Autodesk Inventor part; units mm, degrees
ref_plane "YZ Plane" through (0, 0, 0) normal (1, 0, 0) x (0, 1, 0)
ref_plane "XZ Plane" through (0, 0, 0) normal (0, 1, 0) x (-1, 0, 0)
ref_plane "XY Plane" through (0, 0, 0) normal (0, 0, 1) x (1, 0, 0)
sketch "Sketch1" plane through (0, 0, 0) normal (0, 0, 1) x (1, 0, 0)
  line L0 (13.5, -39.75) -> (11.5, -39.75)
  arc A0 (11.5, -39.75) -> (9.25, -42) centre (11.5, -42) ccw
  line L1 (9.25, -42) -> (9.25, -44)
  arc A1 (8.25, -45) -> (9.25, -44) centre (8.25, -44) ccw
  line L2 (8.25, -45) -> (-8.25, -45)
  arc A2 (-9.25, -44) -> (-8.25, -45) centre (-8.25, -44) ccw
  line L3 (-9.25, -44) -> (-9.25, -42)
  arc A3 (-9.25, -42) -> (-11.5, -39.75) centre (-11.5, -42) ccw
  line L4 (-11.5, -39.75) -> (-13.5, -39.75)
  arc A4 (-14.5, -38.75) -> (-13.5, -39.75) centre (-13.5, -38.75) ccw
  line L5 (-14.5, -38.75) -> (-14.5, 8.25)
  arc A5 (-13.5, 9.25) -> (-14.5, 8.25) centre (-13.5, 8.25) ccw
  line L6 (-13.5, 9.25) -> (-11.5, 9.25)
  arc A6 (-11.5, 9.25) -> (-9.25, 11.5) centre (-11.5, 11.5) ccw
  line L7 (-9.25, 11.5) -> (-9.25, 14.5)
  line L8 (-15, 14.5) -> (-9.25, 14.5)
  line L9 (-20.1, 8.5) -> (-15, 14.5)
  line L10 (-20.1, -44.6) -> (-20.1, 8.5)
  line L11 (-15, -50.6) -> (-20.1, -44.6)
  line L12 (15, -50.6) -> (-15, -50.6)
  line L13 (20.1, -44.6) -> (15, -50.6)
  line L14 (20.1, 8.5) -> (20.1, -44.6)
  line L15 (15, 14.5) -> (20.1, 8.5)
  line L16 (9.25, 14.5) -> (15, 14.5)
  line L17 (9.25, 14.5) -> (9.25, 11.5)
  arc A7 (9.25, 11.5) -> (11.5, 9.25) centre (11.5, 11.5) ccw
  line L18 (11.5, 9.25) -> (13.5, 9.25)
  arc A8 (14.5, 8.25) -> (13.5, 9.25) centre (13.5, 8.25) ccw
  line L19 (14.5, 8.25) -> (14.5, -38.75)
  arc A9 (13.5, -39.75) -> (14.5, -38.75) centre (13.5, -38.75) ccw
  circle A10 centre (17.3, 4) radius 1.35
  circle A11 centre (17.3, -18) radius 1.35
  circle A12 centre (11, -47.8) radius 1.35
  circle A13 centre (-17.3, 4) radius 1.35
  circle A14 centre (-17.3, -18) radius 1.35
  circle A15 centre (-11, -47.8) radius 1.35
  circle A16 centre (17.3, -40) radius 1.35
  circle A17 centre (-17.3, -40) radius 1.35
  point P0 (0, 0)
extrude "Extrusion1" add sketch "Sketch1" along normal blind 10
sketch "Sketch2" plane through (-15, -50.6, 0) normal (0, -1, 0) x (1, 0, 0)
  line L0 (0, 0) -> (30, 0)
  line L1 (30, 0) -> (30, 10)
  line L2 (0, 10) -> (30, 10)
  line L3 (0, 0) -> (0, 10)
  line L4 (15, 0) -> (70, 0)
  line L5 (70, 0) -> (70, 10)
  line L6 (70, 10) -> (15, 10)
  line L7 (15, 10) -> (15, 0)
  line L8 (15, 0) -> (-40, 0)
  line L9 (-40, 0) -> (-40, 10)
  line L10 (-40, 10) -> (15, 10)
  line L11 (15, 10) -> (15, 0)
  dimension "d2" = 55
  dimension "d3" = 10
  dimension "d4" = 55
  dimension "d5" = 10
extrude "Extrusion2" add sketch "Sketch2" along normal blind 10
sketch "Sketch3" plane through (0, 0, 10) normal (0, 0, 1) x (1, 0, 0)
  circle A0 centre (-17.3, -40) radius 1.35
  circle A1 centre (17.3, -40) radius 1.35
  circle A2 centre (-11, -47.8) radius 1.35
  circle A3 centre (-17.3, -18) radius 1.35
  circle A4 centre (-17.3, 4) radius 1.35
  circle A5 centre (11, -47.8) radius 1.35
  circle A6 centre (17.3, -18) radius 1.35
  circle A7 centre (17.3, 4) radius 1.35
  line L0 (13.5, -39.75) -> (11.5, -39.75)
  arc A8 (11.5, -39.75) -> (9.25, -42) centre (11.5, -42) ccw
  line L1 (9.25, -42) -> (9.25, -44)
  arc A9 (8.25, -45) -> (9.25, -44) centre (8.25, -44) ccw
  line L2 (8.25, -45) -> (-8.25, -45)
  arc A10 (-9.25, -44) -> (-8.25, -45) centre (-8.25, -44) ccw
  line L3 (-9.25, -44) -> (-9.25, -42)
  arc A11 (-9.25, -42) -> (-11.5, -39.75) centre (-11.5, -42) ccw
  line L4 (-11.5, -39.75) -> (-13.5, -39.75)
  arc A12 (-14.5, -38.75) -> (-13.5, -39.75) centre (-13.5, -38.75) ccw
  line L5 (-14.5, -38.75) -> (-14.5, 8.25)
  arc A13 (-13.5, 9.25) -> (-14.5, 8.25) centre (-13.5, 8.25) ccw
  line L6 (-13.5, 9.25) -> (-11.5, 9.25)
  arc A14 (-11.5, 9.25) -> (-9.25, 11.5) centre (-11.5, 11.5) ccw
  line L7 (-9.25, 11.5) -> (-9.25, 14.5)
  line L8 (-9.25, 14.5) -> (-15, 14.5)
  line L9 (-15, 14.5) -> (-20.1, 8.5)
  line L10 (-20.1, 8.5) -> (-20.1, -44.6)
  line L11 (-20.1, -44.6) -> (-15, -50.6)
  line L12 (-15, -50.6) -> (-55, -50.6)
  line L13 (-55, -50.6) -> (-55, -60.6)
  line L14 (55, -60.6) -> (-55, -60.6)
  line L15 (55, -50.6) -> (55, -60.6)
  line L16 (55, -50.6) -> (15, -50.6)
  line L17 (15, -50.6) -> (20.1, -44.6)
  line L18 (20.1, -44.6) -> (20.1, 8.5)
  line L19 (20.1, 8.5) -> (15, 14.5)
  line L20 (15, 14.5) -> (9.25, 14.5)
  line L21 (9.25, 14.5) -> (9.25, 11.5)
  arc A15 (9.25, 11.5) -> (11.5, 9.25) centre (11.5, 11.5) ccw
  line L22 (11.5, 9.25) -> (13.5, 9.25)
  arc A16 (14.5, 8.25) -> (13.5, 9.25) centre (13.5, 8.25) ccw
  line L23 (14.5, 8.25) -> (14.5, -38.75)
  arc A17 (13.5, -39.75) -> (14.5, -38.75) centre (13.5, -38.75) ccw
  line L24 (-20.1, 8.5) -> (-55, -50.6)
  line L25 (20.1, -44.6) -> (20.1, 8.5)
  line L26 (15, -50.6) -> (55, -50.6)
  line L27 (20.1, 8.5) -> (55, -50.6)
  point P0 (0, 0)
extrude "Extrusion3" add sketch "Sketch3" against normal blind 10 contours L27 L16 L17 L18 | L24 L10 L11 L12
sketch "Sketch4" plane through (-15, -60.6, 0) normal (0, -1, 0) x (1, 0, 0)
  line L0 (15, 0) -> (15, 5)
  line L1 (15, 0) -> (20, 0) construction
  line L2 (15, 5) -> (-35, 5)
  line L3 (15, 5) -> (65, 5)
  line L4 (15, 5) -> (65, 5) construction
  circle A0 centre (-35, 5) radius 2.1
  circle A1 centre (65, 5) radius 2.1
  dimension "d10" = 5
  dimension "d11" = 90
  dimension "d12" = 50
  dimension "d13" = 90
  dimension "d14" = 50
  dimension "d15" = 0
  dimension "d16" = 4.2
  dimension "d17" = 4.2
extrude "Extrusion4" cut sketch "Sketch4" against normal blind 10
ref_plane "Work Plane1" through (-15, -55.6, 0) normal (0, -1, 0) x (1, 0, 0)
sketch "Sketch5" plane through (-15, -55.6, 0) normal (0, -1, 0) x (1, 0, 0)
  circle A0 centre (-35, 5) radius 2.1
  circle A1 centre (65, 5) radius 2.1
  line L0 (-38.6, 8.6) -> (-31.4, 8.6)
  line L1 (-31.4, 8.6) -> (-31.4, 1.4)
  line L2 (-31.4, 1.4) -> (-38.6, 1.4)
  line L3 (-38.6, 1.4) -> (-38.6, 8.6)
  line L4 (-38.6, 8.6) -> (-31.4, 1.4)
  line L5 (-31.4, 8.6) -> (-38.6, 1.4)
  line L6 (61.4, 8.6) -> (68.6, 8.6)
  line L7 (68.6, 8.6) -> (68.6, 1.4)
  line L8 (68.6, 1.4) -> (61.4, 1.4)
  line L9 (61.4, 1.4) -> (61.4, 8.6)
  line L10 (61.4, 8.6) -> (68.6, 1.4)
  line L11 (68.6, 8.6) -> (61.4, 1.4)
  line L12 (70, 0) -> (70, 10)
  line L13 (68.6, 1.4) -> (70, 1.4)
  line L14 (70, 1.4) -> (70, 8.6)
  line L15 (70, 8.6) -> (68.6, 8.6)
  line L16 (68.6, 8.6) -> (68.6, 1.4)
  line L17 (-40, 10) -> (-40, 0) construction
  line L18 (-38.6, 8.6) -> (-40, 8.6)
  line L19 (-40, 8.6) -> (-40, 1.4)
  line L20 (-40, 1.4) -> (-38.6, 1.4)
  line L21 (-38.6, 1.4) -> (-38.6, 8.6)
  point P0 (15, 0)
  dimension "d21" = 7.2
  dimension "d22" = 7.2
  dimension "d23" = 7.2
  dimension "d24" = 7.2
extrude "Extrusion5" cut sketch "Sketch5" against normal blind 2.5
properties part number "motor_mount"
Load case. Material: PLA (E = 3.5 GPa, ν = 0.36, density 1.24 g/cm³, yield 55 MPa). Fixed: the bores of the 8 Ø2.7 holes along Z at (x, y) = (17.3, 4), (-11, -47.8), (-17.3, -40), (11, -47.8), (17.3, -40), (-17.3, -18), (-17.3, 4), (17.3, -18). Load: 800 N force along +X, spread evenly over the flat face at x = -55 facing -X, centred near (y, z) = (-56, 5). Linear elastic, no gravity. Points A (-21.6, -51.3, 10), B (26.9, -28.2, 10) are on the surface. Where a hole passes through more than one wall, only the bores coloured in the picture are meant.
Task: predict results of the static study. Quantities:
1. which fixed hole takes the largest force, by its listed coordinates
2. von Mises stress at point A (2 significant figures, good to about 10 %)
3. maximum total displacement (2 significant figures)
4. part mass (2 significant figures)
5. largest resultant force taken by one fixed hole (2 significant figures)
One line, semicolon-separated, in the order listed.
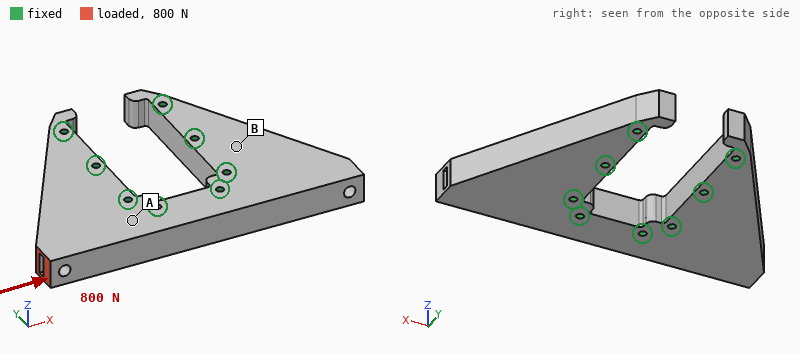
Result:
(-11, -47.8); 4.6 MPa; 0.17 mm; 50 g; 490 N
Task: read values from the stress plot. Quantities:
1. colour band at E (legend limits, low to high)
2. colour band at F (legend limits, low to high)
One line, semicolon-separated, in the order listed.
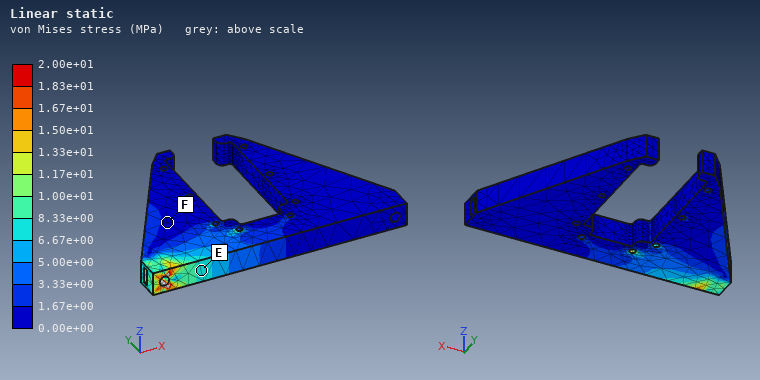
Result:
6.67e+00 to 8.33e+00 MPa; 0.00e+00 to 1.67e+00 MPa
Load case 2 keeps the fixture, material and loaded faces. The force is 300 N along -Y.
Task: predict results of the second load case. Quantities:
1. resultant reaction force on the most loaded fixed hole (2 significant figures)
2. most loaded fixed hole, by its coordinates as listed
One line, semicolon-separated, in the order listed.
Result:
250 N; (-17.3, -18)
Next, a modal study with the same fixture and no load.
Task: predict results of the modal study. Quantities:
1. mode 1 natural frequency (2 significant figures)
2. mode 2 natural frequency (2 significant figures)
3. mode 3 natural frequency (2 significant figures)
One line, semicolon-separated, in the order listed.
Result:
2000 Hz; 2000 Hz; 4900 Hz
